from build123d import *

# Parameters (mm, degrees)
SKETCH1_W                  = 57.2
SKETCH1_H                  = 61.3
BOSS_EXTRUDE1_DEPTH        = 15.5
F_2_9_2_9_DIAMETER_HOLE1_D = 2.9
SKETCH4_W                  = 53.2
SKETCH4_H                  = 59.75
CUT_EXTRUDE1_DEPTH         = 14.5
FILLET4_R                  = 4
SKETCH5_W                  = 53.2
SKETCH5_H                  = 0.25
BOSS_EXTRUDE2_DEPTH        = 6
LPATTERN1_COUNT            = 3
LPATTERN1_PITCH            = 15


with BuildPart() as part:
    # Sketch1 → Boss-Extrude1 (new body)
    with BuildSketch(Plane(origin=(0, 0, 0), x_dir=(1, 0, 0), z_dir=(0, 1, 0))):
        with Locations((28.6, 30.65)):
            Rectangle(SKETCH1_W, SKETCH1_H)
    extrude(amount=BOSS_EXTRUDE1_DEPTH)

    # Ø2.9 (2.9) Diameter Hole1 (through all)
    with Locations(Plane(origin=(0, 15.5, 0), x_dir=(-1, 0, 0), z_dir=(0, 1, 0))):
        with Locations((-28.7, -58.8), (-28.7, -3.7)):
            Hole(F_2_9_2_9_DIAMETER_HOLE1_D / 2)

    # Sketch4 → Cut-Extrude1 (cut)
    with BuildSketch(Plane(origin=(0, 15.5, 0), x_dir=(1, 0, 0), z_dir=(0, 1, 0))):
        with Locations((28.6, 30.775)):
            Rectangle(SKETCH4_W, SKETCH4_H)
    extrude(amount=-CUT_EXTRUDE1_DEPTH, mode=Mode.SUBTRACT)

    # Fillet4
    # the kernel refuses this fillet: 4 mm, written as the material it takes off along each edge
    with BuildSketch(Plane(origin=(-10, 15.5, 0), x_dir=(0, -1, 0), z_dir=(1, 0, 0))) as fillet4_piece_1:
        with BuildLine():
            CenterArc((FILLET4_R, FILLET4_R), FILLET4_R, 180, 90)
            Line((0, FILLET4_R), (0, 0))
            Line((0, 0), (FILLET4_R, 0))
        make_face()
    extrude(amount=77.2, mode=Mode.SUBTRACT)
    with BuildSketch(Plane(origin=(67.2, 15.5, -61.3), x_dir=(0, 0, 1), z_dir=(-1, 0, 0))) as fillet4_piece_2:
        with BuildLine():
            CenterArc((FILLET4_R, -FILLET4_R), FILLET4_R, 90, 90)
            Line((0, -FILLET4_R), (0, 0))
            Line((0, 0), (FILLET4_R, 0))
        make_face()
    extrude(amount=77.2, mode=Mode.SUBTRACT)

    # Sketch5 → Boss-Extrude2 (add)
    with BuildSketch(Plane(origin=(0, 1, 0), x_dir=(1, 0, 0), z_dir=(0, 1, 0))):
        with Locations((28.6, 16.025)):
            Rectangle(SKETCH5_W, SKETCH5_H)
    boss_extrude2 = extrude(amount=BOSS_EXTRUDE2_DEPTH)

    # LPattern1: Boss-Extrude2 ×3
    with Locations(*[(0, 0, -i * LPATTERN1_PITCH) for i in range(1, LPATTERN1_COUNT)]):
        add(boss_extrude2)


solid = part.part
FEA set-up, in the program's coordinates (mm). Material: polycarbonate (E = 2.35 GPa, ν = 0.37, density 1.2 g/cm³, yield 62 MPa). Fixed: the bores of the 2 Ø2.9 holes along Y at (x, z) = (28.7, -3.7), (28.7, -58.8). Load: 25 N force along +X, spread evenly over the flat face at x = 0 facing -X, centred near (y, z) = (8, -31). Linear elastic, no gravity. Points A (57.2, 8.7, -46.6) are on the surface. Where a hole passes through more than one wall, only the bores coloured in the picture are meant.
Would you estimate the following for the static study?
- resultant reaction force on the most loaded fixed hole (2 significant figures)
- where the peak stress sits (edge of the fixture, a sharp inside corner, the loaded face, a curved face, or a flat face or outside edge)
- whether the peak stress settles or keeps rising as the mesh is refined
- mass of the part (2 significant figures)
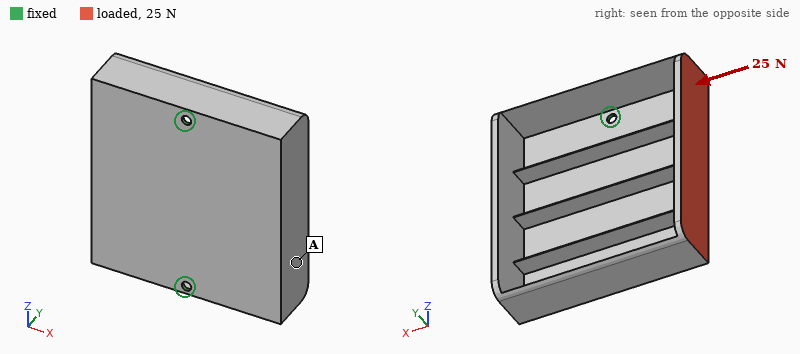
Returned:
13 N
edge of the fixture
keeps rising
9.9 g
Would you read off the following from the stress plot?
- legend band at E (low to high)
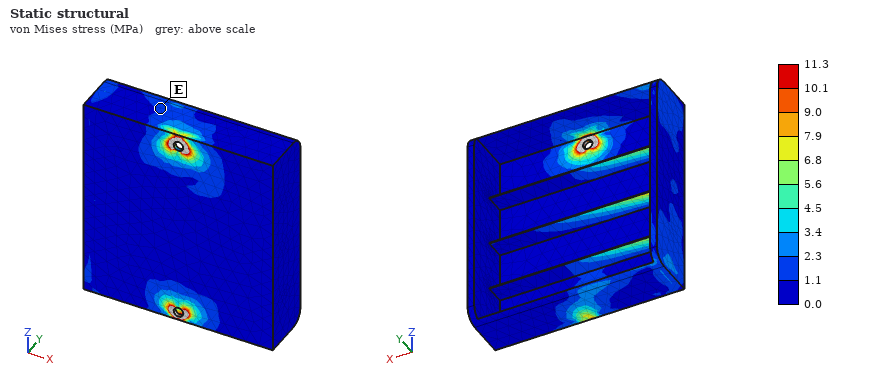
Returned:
1.1 to 2.3 MPa
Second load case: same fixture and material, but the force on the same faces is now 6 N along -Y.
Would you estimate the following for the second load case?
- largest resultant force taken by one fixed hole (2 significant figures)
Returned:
3.1 N
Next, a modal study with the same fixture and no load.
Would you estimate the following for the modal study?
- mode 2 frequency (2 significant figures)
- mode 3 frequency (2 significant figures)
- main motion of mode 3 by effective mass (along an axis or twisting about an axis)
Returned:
370 Hz
820 Hz
along Y
